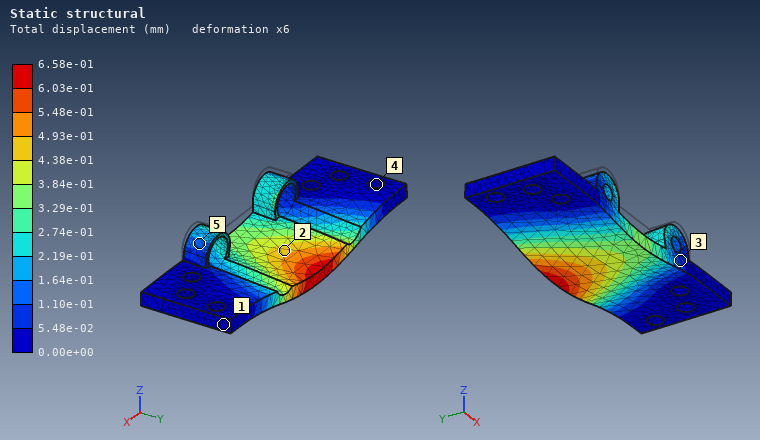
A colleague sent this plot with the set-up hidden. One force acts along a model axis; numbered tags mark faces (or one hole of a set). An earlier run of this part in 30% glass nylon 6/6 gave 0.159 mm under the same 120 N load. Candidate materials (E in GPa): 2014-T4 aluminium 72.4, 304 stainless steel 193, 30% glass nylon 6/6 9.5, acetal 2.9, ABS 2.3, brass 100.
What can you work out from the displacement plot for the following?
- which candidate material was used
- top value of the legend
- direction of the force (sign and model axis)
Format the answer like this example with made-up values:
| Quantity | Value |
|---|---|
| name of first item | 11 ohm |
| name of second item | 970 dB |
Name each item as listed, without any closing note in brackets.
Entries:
| Quantity | Value |
|---|---|
| which candidate material was used | ABS |
| top value of the legend | 6.58e-01 mm |
| direction of the force | -Z |
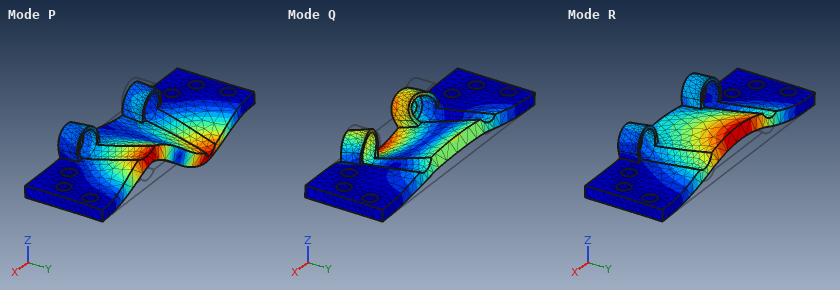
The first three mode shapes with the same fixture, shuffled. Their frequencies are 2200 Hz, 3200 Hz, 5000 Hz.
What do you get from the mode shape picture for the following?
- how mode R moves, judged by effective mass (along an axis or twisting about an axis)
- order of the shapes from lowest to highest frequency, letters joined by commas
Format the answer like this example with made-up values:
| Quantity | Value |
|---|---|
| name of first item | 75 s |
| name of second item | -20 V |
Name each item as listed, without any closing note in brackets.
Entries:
| Quantity | Value |
|---|---|
| how mode R moves, judged by effective mass | along Z |
| order of the shapes from lowest to highest frequency, letters joined by commas | R, Q, P |
